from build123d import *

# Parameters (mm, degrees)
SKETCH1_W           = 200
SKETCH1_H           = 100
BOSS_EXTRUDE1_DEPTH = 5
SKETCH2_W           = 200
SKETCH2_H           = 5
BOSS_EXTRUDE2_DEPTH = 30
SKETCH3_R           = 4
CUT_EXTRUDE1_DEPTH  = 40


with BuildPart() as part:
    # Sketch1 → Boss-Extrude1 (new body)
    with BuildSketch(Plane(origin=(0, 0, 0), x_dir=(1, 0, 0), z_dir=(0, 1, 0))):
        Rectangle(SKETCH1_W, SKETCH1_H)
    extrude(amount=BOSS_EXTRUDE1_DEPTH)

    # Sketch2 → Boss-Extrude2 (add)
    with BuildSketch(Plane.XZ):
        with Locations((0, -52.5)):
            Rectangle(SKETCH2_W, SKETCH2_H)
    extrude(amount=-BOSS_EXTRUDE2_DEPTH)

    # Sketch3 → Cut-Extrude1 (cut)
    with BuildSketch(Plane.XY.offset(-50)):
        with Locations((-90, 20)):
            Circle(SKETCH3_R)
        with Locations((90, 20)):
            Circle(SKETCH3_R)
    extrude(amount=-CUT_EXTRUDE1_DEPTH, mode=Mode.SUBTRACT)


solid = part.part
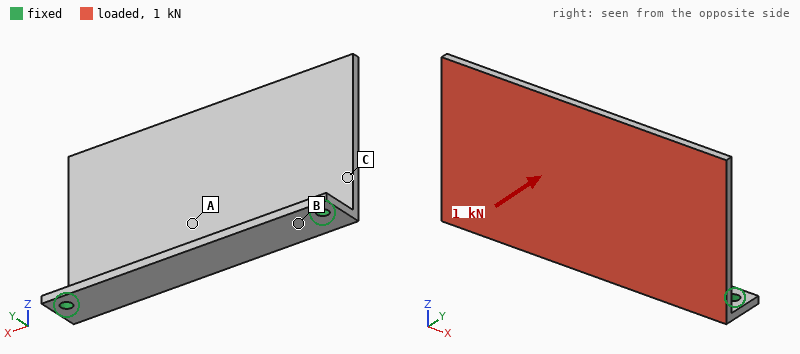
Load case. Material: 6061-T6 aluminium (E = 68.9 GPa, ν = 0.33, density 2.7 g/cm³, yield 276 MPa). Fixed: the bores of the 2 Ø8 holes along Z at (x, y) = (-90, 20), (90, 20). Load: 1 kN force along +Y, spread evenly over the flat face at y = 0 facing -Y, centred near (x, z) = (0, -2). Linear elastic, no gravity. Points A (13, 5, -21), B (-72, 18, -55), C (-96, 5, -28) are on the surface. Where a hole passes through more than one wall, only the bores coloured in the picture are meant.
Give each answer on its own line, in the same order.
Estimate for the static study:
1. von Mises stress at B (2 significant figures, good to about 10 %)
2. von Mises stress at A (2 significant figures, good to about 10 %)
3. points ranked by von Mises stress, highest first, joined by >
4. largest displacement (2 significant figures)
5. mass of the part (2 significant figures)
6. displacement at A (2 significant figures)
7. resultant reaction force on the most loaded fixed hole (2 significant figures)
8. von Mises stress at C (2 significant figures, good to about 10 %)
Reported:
86 MPa
20 MPa
B > C > A
2.6 mm
350 g
0.71 mm
630 N
46 MPa
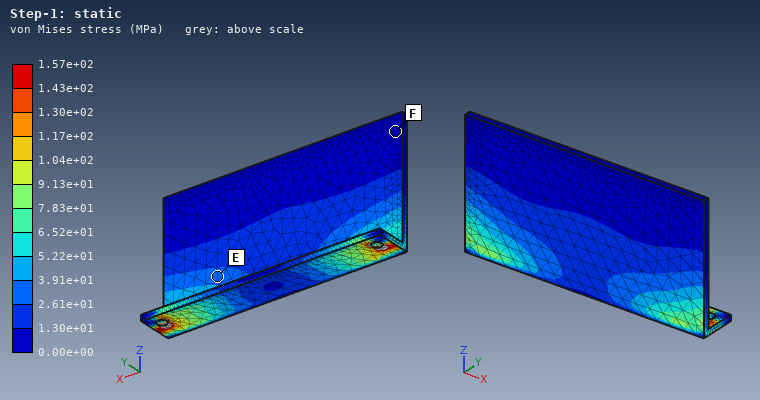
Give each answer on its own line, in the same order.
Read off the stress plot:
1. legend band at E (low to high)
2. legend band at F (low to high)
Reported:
2.61e+01 to 3.91e+01 MPa
0.00e+00 to 1.30e+01 MPa
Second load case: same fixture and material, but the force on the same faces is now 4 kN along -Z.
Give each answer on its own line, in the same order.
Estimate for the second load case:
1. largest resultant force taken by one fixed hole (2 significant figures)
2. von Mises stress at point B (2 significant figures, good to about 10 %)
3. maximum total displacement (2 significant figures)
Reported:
2.0 kN
66 MPa
1.5 mm
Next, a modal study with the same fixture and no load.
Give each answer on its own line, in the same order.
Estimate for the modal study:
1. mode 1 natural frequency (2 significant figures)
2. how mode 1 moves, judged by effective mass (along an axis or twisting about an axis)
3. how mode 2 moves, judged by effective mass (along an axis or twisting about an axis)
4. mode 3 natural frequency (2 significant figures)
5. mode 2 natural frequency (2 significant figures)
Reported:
230 Hz
along Y
twisting about Z
1100 Hz
520 Hz
